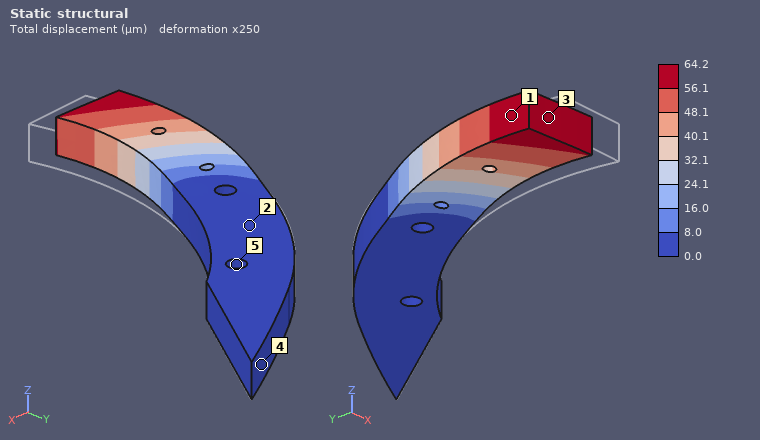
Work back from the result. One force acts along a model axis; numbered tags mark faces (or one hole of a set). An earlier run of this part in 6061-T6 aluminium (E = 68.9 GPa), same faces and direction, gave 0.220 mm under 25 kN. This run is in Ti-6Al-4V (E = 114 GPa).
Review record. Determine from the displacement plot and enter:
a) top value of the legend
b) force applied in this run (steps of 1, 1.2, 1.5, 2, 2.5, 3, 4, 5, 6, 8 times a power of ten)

64.2 µm
12 kN
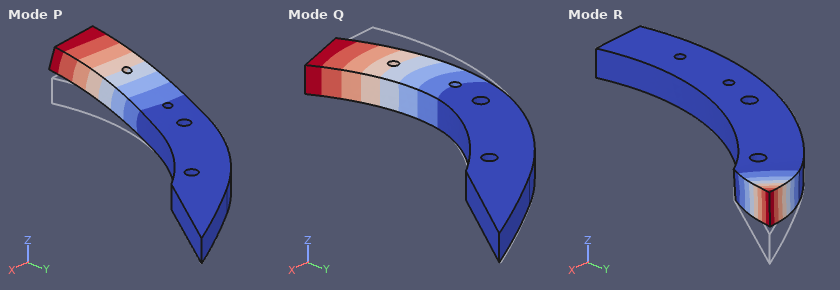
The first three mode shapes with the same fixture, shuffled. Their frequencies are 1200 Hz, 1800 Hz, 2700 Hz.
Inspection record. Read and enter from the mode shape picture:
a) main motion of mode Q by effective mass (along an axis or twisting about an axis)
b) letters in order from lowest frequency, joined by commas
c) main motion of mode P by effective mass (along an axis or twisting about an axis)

along X
P, Q, R
along Z
